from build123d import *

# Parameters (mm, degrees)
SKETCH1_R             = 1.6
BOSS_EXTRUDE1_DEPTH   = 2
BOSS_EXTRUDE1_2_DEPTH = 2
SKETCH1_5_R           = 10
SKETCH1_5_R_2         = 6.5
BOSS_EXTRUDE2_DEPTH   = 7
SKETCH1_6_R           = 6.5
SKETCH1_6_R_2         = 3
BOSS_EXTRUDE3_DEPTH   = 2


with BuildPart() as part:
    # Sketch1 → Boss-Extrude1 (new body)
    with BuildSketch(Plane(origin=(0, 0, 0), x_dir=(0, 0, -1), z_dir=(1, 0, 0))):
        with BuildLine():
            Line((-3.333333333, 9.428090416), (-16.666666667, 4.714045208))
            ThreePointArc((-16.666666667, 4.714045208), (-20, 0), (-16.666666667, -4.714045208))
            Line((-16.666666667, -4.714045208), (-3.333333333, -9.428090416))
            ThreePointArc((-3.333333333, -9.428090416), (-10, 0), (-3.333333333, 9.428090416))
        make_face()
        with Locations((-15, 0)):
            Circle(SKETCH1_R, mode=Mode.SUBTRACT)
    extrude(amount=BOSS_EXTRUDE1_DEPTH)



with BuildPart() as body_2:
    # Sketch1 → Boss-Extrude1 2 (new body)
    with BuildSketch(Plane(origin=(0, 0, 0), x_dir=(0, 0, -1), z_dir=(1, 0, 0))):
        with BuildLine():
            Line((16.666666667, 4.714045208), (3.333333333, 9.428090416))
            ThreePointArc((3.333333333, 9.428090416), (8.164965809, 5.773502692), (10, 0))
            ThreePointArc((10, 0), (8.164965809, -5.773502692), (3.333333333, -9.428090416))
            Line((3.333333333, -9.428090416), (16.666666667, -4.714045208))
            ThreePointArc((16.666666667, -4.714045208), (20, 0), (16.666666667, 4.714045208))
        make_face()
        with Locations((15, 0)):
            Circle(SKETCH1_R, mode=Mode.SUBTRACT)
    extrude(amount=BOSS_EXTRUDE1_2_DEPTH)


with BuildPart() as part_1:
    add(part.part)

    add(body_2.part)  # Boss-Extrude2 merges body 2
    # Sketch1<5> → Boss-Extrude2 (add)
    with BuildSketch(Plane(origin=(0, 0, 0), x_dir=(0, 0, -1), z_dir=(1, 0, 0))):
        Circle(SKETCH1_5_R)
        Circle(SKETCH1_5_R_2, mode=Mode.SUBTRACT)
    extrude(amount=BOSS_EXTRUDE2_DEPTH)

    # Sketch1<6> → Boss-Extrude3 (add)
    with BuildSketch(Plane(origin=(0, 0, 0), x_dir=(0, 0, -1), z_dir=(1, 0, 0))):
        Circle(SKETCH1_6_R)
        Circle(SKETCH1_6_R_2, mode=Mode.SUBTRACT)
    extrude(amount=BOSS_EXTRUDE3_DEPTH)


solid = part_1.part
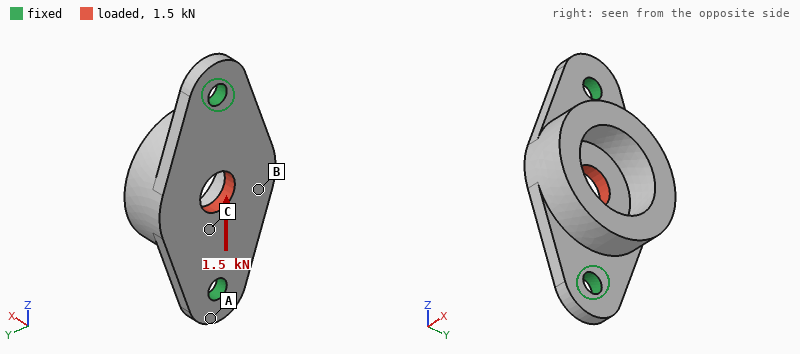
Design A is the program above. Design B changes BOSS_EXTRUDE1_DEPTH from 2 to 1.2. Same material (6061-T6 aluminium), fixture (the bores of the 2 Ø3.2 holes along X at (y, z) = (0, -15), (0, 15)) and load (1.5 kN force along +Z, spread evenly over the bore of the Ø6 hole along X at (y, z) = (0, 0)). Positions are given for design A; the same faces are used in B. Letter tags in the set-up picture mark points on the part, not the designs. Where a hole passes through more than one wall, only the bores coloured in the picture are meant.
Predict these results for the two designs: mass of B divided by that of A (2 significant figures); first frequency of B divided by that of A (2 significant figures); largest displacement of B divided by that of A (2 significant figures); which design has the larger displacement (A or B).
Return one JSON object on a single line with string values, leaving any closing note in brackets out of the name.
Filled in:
{"mass of B divided by that of A": "0.95", "first frequency of B divided by that of A": "0.79", "largest displacement of B divided by that of A": "1.2", "which design has the larger displacement": "B"}
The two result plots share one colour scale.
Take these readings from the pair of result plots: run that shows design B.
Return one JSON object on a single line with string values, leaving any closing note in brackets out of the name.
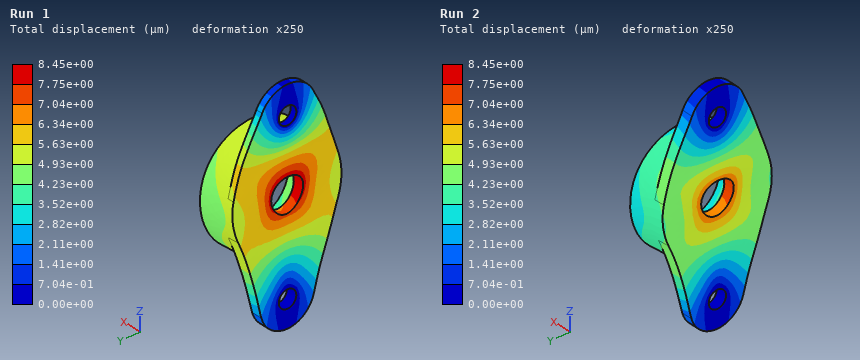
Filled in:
{"run that shows design B": "Run 1"}
